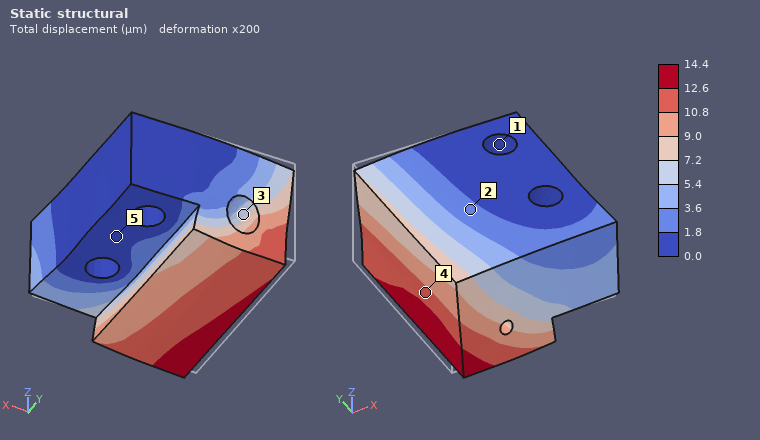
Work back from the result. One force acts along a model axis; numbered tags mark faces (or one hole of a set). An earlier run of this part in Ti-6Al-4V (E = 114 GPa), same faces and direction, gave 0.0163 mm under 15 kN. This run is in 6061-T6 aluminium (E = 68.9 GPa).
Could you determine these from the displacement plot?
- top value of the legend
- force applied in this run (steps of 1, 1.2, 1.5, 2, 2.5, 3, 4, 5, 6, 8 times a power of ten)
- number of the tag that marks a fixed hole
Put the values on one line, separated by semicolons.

14.4 µm; 8 kN; 1
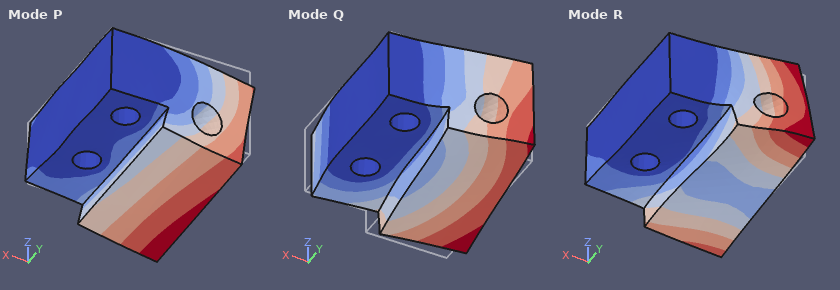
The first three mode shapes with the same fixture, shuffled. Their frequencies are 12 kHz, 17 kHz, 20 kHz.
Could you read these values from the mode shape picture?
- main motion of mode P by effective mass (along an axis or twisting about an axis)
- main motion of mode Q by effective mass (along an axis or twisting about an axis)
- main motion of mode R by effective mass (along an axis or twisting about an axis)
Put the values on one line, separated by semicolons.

along Z; along Y; twisting about X
